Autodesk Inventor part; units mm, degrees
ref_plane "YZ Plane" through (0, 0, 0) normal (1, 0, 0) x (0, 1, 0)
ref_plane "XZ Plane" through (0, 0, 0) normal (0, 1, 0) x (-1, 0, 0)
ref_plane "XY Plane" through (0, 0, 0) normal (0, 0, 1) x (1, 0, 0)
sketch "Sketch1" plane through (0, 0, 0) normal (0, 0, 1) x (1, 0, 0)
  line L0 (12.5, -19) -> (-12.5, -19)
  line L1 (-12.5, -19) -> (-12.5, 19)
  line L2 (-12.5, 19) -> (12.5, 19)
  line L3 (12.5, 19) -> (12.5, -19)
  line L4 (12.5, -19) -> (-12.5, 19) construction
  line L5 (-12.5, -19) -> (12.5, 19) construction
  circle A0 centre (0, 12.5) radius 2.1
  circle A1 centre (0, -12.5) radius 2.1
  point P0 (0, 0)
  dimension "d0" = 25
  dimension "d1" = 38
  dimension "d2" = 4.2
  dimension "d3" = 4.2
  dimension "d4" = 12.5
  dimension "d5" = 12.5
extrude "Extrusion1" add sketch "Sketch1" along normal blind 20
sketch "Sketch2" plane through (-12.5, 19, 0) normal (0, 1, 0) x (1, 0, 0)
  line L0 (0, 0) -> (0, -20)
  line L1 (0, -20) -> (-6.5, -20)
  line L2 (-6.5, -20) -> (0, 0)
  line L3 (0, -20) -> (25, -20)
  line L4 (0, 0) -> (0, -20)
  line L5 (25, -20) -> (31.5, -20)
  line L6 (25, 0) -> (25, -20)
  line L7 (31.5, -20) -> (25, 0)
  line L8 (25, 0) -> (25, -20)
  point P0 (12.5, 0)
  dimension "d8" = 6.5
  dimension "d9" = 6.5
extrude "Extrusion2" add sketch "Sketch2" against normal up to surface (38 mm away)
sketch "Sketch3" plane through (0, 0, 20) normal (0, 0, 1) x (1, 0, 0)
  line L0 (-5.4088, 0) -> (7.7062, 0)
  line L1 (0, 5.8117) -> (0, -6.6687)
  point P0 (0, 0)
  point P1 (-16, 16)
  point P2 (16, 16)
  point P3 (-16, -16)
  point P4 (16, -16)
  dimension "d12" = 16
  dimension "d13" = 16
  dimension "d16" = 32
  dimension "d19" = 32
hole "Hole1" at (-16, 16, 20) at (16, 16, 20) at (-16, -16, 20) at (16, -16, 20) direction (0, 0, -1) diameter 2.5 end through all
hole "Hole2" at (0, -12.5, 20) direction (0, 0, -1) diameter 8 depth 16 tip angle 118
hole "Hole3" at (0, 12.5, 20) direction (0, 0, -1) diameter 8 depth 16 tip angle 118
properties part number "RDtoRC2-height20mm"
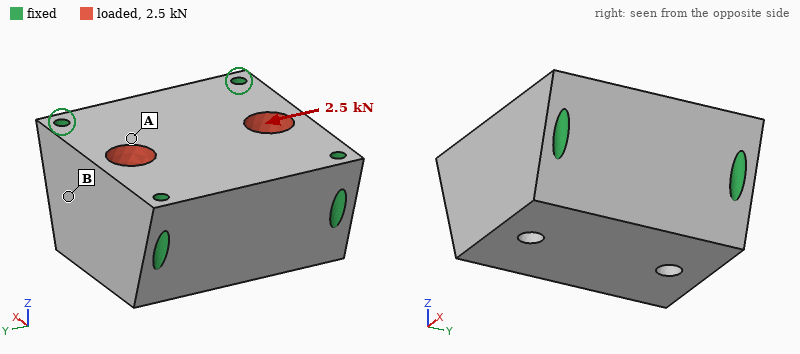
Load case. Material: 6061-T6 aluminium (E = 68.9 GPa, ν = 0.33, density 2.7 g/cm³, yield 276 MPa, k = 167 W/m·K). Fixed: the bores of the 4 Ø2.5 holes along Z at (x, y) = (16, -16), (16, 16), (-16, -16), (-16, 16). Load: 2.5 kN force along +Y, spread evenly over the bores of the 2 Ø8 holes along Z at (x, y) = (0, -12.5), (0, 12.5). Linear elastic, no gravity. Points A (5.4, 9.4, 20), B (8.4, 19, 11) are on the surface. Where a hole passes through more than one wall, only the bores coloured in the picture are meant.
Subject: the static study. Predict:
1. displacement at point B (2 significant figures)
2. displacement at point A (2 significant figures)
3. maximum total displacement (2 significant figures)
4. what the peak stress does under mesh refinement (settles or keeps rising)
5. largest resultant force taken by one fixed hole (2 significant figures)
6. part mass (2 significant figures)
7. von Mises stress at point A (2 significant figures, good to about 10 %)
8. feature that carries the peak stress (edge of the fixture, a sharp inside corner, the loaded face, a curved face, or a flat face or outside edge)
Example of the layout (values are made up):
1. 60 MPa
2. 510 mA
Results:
1. 1.5 µm
2. 1.7 µm
3. 3.0 µm
4. keeps rising
5. 680 N
6. 59 g
7. 6.1 MPa
8. edge of the fixture
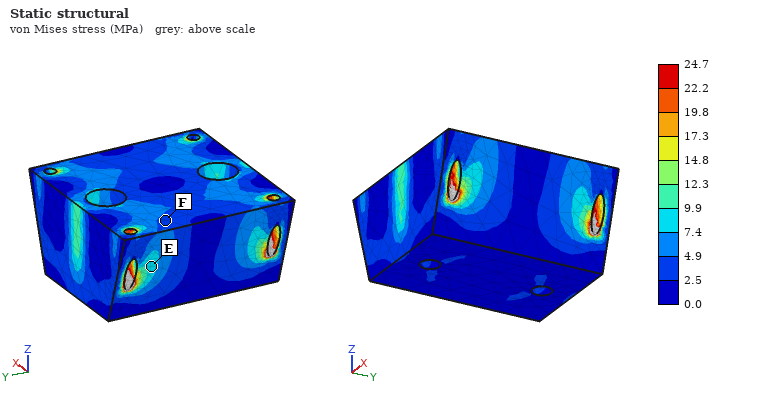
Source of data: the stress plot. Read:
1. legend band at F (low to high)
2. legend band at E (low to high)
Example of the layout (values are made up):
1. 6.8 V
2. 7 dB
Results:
1. 2.5 to 4.9 MPa
2. 7.4 to 9.9 MPa
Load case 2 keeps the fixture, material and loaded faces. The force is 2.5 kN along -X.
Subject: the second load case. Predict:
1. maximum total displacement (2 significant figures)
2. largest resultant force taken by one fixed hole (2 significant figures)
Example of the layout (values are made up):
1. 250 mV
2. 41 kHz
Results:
1. 1.3 µm
2. 650 N
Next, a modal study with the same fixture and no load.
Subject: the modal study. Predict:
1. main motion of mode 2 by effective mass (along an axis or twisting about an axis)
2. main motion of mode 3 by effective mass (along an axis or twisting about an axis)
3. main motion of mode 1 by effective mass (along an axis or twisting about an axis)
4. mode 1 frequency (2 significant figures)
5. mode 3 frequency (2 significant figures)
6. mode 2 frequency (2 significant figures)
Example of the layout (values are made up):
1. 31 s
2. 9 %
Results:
1. along Y
2. along X
3. along Z
4. 24 kHz
5. 30 kHz
6. 29 kHz
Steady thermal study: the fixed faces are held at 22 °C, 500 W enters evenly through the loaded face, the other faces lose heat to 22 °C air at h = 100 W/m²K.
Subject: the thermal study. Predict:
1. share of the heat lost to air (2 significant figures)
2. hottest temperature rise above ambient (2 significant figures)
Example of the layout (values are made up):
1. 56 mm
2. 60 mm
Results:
1. 3.8 %
2. 63 K
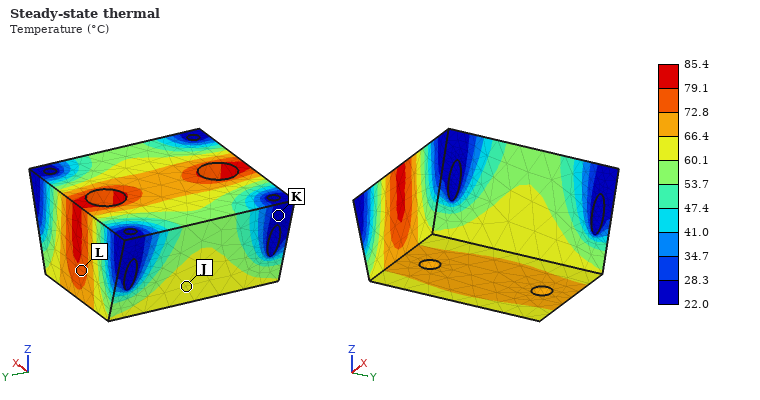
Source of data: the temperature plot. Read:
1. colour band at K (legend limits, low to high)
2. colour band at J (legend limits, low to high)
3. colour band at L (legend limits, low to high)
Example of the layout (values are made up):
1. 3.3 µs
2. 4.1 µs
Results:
1. 22.0 to 28.3 °C
2. 60.1 to 66.4 °C
3. 72.8 to 79.1 °C
